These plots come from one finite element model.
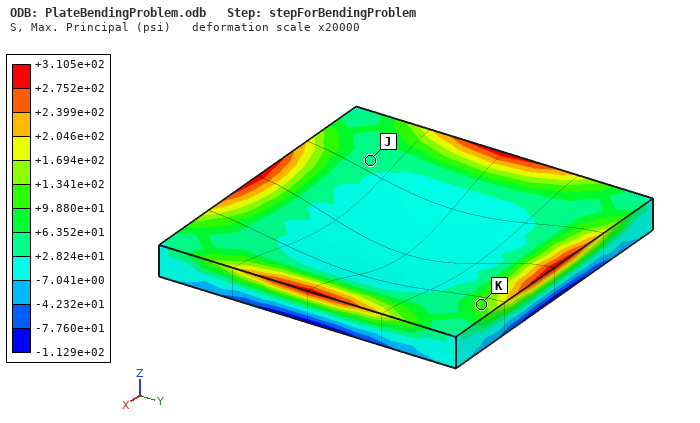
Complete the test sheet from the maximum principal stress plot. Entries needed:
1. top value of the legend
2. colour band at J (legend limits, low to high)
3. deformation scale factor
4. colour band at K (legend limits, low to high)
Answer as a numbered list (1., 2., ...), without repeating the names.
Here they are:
1. +3.105e+02 psi
2. +2.824e+01 to +6.352e+01 psi
3. 20000
4. +9.880e+01 to +1.341e+02 psi
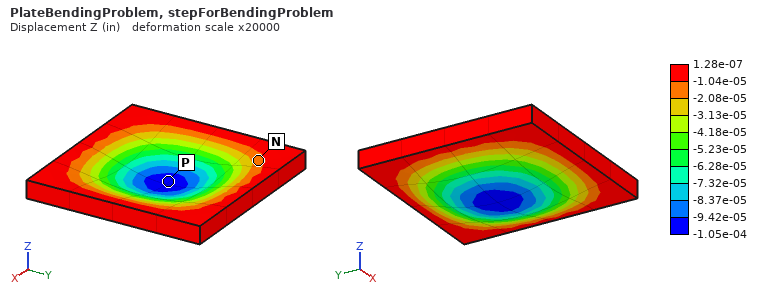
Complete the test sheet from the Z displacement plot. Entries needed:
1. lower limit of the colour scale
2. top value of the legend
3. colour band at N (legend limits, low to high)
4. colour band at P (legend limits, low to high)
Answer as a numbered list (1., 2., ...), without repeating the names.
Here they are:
1. -1.05e-04 in
2. 1.28e-07 in
3. -2.08e-05 to -1.04e-05 in
4. -1.05e-04 to -9.42e-05 in
